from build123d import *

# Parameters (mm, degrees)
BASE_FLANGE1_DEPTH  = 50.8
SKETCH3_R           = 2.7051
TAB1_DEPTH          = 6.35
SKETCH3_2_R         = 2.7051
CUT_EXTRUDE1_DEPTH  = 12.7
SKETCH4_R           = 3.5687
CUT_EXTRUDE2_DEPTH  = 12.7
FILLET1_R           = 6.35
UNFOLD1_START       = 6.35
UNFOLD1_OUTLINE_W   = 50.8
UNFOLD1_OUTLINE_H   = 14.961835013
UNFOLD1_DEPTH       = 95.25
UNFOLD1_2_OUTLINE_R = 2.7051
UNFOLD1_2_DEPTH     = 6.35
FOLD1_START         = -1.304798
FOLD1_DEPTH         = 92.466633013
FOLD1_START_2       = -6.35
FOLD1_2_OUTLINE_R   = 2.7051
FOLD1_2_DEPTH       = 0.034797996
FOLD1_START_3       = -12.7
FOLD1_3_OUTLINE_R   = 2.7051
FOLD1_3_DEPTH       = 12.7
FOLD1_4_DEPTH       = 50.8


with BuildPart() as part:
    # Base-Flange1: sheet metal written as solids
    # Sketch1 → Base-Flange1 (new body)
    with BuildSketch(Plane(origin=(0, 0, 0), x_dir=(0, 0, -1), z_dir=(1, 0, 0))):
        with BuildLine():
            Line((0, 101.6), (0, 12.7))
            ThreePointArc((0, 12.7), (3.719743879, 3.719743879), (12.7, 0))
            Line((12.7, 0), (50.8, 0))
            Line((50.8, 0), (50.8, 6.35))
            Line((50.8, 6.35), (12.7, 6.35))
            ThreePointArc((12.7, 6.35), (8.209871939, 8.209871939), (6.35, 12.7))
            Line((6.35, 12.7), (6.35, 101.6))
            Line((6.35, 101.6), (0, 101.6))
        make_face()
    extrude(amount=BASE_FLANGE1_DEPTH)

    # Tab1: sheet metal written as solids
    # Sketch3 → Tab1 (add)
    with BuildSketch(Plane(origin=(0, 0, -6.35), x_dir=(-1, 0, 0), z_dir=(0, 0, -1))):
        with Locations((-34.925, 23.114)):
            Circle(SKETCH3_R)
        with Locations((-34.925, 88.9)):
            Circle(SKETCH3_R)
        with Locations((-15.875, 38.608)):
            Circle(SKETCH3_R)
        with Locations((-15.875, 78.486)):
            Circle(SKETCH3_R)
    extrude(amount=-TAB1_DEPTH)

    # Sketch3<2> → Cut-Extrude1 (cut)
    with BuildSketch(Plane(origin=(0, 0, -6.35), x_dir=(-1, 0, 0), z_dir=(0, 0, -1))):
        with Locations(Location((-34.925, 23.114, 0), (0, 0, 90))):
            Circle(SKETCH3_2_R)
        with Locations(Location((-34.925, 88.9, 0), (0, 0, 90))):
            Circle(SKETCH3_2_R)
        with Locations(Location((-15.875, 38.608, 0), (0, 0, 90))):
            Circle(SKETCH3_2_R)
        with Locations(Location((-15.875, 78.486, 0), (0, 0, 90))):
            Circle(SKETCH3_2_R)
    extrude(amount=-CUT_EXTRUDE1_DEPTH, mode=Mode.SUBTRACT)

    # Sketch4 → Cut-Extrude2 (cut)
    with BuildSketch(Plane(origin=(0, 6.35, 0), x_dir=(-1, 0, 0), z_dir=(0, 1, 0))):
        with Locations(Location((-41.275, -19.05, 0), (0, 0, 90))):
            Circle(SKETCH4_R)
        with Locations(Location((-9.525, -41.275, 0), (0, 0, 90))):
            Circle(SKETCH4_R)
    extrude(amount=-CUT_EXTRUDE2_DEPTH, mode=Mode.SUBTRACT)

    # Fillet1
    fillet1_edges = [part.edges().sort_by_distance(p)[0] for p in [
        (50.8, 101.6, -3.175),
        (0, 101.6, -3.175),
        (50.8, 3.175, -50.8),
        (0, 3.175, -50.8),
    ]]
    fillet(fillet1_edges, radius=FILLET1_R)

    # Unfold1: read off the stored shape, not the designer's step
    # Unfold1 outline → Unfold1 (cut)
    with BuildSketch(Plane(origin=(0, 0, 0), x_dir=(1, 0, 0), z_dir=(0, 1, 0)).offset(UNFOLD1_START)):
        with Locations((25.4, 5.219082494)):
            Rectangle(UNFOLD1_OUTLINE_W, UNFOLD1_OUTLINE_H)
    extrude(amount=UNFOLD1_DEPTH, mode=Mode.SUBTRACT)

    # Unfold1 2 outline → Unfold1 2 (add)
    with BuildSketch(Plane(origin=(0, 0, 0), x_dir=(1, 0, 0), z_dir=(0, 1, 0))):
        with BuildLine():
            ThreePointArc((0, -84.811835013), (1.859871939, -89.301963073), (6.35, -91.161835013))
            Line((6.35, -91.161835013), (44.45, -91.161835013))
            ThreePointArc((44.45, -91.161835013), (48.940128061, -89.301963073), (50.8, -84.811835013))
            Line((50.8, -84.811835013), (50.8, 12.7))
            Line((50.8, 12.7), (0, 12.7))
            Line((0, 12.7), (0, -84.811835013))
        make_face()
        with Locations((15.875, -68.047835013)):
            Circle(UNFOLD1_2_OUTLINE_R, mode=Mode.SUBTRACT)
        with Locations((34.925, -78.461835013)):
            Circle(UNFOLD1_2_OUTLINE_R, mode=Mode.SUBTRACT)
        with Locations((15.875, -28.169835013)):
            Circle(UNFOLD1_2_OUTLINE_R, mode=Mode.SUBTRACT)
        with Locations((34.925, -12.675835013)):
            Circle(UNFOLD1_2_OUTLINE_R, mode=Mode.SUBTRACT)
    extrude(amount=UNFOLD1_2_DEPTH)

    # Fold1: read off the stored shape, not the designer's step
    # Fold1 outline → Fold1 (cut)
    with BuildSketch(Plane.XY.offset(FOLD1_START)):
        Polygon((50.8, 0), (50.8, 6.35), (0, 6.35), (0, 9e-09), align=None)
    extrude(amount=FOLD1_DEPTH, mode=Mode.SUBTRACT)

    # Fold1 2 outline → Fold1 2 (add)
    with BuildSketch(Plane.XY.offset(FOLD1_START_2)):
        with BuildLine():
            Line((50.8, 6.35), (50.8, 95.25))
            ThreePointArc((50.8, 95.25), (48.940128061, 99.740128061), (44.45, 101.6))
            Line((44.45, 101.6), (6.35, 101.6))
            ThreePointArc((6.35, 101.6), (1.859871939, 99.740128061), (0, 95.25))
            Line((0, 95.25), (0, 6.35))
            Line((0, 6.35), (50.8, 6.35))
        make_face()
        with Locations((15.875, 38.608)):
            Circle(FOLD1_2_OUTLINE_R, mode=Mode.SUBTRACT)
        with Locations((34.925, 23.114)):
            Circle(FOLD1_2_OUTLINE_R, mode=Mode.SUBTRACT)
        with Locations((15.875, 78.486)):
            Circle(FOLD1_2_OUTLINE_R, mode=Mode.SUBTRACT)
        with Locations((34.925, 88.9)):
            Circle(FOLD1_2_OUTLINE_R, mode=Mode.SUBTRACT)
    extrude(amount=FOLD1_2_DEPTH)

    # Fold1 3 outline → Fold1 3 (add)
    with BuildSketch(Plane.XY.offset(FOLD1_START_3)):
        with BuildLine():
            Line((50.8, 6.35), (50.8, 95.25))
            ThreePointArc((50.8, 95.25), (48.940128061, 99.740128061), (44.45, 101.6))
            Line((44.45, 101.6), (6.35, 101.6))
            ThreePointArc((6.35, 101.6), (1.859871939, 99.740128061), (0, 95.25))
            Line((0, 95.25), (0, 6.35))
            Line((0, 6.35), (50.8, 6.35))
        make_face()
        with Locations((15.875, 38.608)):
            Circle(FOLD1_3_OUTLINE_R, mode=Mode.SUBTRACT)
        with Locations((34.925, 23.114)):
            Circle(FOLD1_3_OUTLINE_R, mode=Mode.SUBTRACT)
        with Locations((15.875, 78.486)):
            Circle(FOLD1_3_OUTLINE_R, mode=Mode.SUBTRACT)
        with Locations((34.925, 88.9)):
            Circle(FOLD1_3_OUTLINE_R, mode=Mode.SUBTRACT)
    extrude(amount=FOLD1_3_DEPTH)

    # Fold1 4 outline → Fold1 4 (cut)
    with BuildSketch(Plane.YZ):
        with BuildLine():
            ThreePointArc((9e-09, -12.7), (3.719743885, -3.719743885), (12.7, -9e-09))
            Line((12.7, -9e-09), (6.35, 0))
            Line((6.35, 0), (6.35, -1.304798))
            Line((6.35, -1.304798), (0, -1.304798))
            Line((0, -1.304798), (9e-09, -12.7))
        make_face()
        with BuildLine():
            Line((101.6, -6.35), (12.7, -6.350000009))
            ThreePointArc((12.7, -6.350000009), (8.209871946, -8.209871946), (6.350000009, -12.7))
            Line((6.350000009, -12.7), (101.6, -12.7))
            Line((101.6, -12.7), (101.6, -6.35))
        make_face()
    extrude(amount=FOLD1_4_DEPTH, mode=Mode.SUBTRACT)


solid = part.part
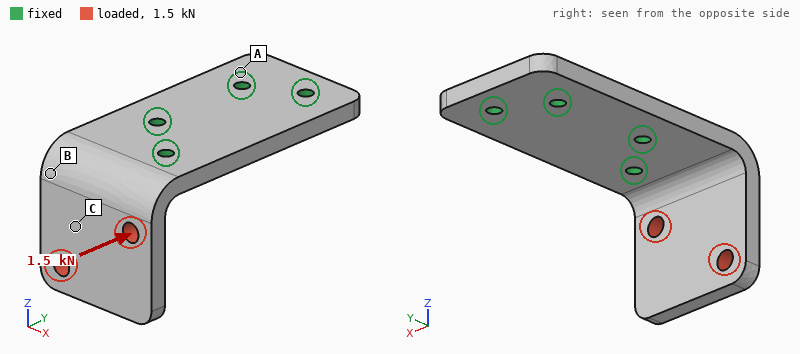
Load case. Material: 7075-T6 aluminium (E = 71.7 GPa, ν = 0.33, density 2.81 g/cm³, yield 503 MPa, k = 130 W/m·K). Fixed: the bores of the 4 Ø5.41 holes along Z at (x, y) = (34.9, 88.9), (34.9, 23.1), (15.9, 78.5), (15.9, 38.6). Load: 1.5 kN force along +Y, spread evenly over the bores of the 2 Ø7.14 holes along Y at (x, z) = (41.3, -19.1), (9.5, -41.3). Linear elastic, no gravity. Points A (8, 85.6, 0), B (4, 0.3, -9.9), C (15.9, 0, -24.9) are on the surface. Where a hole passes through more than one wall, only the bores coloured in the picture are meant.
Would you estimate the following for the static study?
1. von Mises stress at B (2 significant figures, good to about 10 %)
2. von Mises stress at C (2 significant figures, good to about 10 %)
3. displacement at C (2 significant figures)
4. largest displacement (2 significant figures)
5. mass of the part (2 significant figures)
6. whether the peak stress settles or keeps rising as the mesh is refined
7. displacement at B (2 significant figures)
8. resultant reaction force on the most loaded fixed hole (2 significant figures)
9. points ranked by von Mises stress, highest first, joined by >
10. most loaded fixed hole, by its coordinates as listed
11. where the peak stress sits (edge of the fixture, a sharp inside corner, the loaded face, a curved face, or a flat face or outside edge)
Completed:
71 MPa
43 MPa
0.37 mm
0.82 mm
120 g
keeps rising
0.23 mm
1.0 kN
B > C > A
(34.9, 23.1)
edge of the fixture
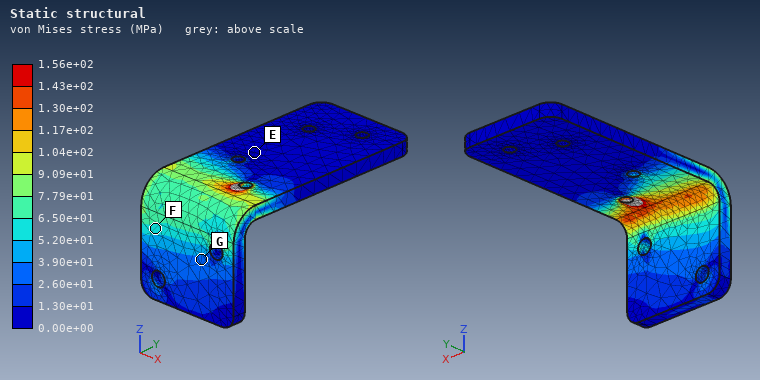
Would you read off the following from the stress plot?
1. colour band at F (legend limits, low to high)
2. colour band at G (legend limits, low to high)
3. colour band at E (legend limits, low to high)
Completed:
5.20e+01 to 6.50e+01 MPa
2.60e+01 to 3.90e+01 MPa
0.00e+00 to 1.30e+01 MPa
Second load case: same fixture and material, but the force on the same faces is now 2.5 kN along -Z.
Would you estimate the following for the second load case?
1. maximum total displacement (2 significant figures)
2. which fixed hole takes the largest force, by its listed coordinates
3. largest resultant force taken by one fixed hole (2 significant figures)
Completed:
0.51 mm
(34.9, 23.1)
2.5 kN
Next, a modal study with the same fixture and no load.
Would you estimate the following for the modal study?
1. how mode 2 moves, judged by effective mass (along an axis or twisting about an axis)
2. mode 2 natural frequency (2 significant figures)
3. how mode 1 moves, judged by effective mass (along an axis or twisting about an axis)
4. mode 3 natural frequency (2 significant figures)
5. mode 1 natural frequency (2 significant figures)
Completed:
along X
2100 Hz
along Y
4600 Hz
1400 Hz
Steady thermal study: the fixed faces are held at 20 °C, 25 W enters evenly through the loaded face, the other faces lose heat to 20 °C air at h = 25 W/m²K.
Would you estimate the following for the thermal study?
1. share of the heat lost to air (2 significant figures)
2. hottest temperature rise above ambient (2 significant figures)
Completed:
14 %
32 K
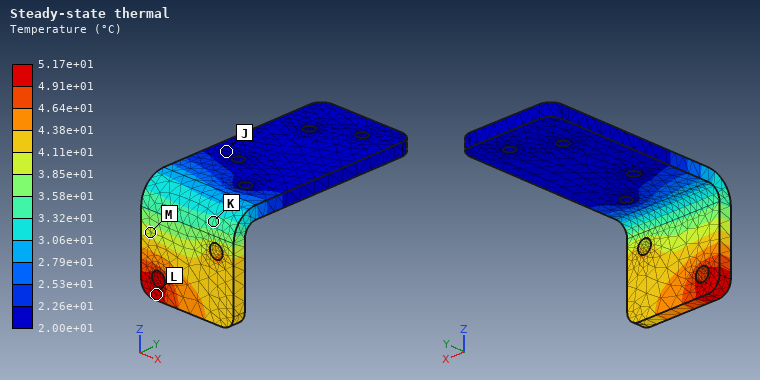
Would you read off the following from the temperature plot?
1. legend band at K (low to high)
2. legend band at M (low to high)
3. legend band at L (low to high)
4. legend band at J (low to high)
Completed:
3.32e+01 to 3.58e+01 °C
3.85e+01 to 4.11e+01 °C
4.91e+01 to 5.17e+01 °C
2.00e+01 to 2.26e+01 °C
